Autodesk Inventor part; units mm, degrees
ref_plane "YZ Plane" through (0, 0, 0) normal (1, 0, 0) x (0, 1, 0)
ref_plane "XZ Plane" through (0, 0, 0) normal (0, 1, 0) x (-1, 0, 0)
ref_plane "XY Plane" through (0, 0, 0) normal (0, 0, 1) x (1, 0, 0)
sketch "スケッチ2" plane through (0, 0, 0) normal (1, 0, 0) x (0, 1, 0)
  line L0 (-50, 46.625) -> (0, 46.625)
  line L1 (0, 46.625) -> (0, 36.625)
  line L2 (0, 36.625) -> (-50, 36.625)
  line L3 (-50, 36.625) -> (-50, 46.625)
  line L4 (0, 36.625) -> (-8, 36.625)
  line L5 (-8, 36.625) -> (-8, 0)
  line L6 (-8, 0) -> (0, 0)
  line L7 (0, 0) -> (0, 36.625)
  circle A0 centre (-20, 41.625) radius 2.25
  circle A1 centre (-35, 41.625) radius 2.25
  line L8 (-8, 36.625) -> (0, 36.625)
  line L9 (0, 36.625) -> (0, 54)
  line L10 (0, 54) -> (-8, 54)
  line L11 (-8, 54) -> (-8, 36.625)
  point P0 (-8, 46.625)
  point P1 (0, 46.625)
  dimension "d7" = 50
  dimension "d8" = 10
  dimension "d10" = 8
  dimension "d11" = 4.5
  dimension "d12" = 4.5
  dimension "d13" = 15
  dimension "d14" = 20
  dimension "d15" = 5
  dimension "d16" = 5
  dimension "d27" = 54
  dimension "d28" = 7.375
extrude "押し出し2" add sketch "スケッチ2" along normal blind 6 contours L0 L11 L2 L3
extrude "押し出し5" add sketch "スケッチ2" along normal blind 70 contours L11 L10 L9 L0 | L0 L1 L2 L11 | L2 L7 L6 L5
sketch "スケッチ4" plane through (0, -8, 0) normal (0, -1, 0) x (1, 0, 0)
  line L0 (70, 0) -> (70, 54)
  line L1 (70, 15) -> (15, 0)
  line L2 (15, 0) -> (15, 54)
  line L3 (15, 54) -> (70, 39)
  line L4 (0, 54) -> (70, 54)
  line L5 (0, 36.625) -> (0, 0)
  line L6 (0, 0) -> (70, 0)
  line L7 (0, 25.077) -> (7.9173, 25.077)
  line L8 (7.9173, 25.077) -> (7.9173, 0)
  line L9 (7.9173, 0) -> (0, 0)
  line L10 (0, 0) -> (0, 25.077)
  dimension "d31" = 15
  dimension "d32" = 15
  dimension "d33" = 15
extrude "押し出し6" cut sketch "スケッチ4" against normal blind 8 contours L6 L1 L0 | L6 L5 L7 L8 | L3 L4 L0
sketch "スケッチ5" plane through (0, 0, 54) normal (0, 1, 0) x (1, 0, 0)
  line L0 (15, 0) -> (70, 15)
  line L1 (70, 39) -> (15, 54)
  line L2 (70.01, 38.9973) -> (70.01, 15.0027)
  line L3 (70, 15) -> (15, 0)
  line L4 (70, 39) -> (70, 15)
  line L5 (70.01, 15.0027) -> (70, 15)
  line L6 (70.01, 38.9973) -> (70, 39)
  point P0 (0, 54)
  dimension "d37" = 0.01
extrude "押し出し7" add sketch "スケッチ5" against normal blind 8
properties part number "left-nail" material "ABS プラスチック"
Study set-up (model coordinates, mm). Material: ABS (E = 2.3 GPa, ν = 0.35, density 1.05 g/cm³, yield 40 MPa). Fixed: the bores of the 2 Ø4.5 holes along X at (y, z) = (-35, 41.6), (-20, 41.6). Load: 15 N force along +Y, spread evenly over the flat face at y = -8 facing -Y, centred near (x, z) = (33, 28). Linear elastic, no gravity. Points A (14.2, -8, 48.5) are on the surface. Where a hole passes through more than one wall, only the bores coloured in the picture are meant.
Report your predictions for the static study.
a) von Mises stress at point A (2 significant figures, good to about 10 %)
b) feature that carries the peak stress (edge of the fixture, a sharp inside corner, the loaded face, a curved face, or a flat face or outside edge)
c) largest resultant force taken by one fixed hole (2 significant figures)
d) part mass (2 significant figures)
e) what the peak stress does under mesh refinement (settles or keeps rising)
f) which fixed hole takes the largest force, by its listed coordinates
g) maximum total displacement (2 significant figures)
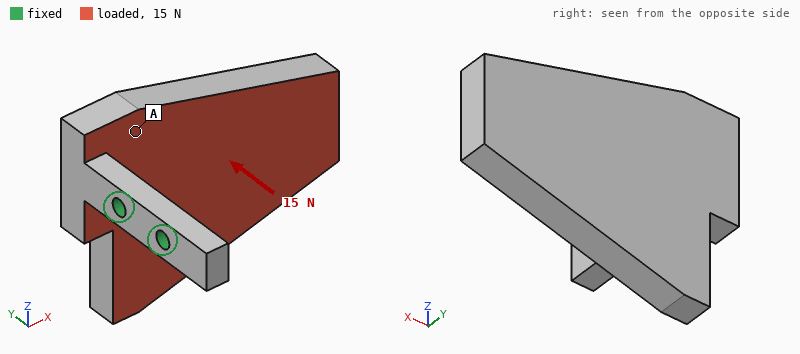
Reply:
1.0 MPa
edge of the fixture
15 N
26 g
keeps rising
(-20, 41.6)
1.2 mm
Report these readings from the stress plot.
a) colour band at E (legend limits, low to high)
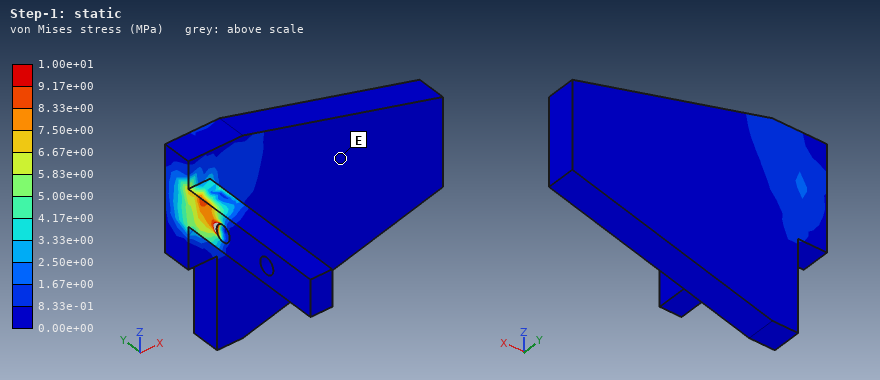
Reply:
0.00e+00 to 8.33e-01 MPa
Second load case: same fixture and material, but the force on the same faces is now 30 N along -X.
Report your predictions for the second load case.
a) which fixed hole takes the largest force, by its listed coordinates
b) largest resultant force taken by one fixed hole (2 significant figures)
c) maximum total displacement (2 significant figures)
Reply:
(-20, 41.6)
32 N
0.95 mm
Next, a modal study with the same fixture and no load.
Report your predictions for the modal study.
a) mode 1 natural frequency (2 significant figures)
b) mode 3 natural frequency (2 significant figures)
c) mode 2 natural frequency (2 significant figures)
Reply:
150 Hz
520 Hz
160 Hz
